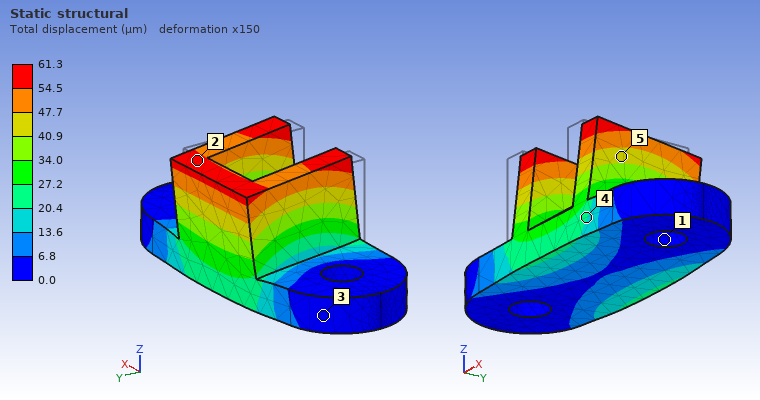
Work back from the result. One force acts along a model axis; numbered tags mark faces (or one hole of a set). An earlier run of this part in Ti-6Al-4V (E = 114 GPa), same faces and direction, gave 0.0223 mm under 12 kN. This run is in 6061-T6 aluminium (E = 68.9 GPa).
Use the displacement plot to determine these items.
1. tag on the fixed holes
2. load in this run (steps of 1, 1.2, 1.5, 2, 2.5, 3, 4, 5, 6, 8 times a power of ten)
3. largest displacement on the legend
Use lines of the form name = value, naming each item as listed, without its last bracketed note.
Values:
tag on the fixed holes = 1
load in this run = 20 kN
largest displacement on the legend = 61.3 µm
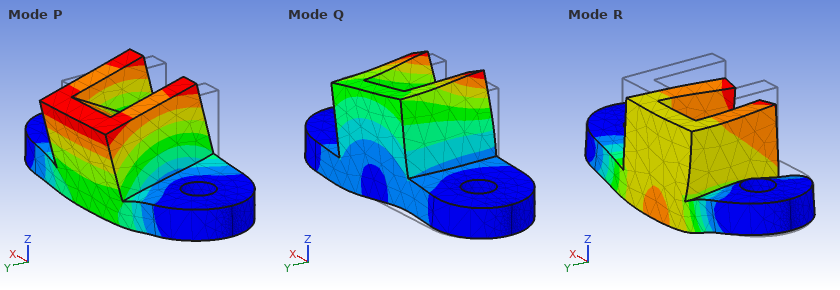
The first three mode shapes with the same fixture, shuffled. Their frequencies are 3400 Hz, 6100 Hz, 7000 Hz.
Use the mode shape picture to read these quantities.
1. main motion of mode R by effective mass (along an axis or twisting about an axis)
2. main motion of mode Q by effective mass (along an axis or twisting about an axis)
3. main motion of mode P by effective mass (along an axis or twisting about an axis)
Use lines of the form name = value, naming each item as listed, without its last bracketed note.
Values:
main motion of mode R by effective mass = along Z
main motion of mode Q by effective mass = along X
main motion of mode P by effective mass = along Y
